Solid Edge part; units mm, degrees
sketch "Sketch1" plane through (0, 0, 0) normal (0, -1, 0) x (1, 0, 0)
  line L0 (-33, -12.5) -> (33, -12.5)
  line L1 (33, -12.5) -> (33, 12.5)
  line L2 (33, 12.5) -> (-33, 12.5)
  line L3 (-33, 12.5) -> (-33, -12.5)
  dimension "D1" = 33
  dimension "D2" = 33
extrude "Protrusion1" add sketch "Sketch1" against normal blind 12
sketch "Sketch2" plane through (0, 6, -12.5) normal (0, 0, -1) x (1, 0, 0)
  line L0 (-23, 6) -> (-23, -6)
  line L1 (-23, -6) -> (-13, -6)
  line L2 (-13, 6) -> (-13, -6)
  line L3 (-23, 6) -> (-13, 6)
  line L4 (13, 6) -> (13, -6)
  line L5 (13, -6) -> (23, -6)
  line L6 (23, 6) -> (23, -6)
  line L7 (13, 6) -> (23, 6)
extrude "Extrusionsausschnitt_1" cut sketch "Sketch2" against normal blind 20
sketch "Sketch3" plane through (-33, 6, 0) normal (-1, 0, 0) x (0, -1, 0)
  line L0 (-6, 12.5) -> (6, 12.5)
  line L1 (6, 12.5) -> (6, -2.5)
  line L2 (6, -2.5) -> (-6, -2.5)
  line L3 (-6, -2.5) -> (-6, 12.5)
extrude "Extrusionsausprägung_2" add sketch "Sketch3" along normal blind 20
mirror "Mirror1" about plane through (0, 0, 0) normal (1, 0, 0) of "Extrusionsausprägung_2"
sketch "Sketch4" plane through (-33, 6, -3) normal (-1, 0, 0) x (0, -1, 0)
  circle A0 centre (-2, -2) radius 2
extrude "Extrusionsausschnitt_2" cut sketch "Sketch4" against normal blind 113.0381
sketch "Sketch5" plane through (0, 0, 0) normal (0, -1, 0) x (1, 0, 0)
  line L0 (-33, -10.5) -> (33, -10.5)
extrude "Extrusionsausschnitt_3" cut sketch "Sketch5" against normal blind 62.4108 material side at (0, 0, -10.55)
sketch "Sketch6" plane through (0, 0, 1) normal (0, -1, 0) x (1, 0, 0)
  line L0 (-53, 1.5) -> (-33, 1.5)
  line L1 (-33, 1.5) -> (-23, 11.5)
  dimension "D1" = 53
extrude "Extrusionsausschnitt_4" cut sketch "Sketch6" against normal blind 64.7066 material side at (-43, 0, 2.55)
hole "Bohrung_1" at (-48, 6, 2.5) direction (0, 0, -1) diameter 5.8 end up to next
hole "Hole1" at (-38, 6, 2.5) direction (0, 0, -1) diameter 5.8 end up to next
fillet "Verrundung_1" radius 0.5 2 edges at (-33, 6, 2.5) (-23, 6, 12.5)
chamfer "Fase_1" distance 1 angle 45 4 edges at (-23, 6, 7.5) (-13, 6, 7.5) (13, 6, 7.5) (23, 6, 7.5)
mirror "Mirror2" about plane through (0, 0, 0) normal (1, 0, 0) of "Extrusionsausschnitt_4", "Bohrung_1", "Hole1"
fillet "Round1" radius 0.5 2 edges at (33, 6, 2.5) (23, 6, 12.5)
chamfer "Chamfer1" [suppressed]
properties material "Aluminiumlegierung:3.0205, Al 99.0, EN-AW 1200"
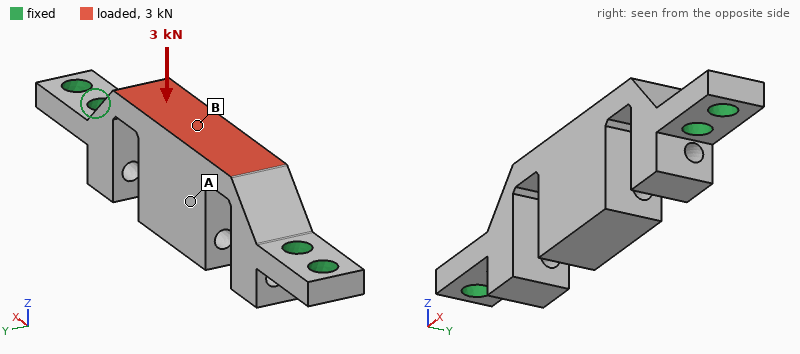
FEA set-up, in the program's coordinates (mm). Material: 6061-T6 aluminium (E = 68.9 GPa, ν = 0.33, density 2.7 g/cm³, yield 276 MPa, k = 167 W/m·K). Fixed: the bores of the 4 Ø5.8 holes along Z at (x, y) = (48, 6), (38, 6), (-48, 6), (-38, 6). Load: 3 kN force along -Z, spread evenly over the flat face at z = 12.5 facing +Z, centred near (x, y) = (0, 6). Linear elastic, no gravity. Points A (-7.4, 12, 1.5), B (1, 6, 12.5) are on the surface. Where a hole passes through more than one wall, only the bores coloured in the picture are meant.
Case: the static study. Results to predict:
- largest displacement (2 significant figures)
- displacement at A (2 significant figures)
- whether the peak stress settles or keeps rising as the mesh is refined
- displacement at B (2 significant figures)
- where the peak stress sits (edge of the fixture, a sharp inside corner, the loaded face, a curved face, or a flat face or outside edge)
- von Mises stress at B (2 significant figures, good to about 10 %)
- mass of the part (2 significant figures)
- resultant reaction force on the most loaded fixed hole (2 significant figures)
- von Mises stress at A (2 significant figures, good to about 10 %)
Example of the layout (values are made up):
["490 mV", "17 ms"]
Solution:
["89 µm", "86 µm", "keeps rising", "88 µm", "edge of the fixture", "51 MPa", "38 g", "2.4 kN", "20 MPa"]
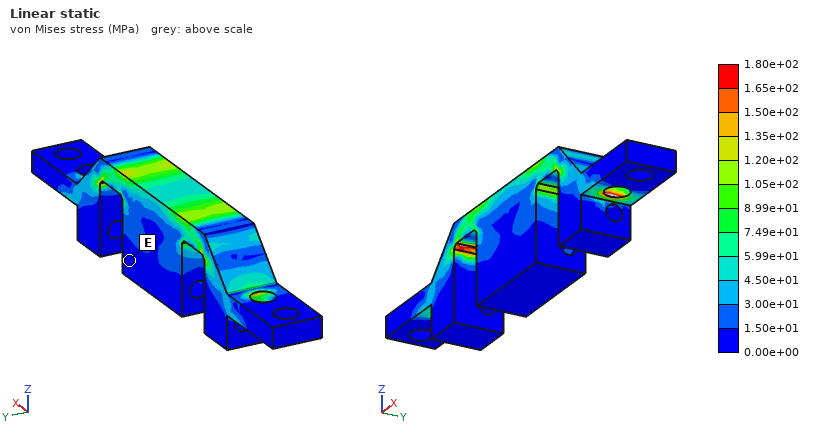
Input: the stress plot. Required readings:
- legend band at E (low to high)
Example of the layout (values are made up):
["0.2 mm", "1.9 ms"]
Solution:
["0.00e+00 to 1.50e+01 MPa"]
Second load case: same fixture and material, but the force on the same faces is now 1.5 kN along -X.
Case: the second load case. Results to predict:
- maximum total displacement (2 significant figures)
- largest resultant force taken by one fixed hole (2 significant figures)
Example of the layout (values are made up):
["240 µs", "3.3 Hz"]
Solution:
["51 µm", "730 N"]
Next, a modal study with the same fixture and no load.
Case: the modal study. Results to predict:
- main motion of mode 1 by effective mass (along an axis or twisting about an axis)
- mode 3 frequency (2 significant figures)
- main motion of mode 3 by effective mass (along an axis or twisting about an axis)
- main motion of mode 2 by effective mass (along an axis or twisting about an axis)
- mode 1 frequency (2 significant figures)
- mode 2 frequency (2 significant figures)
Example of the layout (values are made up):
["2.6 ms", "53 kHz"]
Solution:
["along Y", "6000 Hz", "along Z", "along X", "3400 Hz", "4500 Hz"]
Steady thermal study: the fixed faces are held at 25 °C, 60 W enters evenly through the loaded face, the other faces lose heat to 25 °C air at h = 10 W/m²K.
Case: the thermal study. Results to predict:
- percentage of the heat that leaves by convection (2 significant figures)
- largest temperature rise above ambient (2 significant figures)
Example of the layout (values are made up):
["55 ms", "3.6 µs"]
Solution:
["3.7 %", "73 K"]
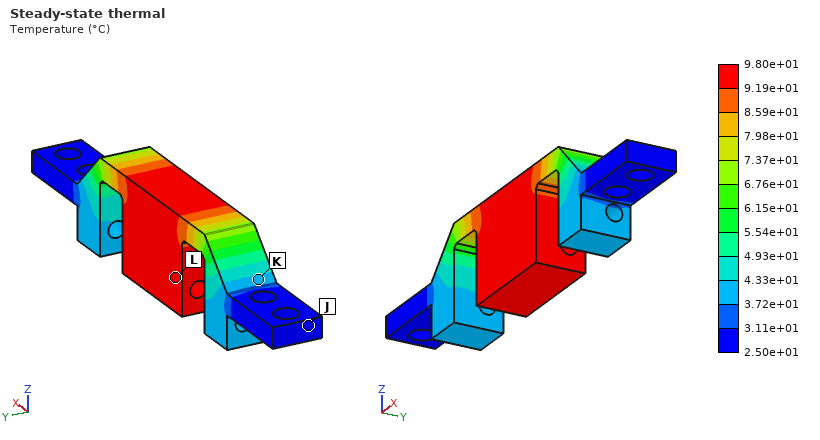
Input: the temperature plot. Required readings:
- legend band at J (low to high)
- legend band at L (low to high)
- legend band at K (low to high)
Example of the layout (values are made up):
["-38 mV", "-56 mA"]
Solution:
["2.50e+01 to 3.11e+01 °C", "9.19e+01 to 9.80e+01 °C", "3.72e+01 to 4.33e+01 °C"]
